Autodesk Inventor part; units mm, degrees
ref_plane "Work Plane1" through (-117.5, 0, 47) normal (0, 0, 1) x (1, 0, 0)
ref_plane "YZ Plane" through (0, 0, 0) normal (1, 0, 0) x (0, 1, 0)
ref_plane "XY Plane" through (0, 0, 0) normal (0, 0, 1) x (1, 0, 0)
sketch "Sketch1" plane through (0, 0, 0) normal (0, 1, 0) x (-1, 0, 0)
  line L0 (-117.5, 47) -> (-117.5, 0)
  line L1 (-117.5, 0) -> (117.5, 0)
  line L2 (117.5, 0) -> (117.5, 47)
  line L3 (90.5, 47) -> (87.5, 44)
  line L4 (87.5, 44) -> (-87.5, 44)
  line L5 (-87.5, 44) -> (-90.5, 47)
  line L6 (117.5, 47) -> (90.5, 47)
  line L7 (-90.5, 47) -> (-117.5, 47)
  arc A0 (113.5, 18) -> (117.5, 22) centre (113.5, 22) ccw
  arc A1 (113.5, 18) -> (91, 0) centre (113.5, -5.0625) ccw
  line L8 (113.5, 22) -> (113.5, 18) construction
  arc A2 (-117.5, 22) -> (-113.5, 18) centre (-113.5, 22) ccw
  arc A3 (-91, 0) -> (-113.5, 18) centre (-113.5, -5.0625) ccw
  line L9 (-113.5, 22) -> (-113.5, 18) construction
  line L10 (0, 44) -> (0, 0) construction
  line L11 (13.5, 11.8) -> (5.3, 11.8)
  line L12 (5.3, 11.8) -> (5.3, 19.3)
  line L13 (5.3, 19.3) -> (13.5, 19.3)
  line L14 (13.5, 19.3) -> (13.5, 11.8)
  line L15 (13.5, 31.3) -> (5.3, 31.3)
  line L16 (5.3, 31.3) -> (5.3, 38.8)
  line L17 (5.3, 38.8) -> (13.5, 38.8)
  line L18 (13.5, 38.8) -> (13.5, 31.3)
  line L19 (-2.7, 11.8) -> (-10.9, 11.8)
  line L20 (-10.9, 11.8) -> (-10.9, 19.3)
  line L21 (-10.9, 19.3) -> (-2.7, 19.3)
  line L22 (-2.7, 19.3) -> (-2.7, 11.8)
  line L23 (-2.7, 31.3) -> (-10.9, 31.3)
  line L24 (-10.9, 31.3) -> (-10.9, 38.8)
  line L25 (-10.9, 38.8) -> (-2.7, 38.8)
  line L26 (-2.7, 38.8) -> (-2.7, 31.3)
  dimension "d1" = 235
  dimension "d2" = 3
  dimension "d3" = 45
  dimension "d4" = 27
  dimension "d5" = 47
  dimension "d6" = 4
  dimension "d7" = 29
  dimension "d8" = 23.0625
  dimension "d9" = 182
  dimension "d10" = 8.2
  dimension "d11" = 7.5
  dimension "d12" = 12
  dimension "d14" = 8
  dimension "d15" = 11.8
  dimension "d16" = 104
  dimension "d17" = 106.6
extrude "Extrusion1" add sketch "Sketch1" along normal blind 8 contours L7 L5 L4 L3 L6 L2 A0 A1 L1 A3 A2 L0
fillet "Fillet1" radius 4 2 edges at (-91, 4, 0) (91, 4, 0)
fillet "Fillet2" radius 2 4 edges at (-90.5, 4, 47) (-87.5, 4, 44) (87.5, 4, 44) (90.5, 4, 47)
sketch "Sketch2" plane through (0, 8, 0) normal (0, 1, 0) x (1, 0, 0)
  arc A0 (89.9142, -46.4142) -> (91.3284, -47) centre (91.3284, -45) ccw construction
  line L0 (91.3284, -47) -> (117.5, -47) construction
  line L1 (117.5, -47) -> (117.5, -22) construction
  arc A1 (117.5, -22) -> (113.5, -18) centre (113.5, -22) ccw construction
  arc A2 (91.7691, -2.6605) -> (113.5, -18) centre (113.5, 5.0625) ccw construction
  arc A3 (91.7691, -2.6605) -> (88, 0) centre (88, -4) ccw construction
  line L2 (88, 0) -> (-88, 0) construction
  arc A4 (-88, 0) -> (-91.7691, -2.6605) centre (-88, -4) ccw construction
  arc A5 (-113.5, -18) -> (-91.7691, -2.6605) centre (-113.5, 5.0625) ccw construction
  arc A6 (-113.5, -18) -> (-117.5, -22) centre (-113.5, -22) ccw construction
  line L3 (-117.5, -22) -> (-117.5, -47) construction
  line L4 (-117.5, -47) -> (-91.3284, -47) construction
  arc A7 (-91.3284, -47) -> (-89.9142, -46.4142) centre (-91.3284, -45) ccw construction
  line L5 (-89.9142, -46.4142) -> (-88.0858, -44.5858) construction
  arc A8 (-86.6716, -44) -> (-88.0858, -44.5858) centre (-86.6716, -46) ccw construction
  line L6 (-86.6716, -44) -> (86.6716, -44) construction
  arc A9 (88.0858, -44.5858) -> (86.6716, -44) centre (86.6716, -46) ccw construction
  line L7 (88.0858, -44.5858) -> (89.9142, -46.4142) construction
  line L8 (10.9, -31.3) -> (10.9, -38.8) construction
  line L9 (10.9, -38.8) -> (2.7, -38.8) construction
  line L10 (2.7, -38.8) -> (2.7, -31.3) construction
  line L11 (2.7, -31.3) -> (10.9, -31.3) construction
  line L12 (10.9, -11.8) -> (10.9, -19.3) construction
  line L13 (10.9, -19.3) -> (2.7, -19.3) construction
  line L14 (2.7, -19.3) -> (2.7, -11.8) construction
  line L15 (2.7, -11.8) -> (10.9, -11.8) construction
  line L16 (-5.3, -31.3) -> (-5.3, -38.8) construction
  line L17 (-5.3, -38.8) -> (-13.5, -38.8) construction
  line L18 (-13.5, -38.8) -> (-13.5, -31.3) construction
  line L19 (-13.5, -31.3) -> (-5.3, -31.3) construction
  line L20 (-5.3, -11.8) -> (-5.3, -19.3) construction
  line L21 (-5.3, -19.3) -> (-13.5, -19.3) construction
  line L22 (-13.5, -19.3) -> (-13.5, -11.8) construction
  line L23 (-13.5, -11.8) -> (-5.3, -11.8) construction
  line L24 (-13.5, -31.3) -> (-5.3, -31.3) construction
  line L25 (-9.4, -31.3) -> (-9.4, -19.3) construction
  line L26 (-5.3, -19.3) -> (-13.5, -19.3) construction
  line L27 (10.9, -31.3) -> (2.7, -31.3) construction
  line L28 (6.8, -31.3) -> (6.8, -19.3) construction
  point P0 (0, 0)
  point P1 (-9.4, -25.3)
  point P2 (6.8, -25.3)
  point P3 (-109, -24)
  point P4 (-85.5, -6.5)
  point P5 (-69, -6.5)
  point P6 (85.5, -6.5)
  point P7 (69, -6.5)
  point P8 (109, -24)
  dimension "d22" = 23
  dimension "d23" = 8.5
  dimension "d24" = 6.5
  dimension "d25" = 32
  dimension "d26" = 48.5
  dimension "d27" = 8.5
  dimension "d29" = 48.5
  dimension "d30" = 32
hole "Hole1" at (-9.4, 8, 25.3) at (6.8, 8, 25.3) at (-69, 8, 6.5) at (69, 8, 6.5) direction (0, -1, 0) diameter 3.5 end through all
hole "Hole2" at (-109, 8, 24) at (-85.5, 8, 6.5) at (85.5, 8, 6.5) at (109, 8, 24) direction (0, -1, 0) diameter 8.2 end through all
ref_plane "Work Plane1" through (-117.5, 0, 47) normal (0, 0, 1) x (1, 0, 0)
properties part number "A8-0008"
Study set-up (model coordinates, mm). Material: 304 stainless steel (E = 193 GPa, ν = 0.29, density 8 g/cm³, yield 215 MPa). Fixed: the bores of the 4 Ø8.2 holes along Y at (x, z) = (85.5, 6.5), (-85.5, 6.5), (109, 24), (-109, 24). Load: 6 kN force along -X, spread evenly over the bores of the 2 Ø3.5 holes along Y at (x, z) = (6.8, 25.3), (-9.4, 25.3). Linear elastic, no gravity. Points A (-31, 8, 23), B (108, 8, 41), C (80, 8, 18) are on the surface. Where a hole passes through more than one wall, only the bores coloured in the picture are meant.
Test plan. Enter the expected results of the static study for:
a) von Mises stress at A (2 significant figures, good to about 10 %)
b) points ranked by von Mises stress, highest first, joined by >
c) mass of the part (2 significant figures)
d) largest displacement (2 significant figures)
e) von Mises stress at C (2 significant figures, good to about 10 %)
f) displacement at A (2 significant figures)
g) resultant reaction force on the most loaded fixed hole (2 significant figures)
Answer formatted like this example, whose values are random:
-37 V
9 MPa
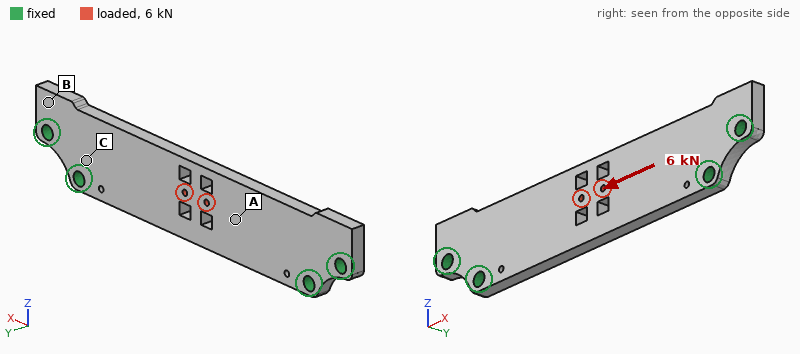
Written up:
13 MPa
A > C > B
590 g
6.0 µm
7.5 MPa
3.3 µm
1.8 kN
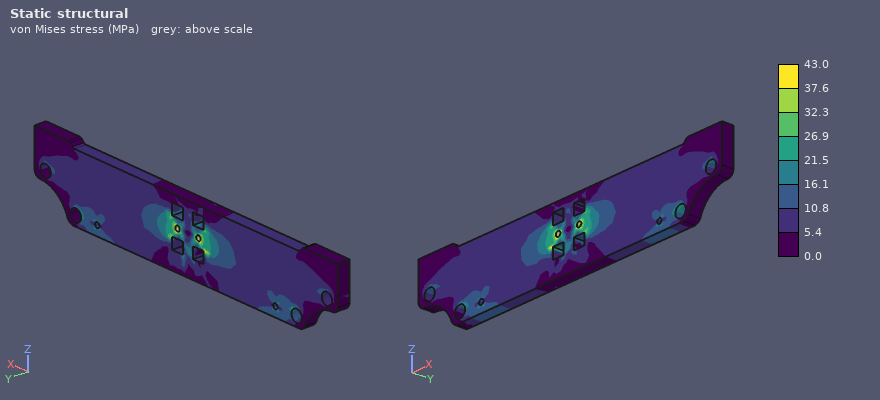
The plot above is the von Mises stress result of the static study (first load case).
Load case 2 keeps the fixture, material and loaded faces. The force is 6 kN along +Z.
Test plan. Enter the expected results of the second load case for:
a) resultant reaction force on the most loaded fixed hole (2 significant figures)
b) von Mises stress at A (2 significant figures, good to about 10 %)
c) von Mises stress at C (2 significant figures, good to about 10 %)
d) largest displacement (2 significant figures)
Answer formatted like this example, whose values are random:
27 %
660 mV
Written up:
5.8 kN
20 MPa
23 MPa
34 µm
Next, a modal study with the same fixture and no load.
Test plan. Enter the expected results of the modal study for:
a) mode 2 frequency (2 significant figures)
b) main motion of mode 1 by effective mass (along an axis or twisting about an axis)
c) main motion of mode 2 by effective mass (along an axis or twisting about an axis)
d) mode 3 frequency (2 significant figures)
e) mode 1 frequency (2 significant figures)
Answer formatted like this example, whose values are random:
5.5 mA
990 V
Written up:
3000 Hz
along Y
twisting about X
3200 Hz
1200 Hz
